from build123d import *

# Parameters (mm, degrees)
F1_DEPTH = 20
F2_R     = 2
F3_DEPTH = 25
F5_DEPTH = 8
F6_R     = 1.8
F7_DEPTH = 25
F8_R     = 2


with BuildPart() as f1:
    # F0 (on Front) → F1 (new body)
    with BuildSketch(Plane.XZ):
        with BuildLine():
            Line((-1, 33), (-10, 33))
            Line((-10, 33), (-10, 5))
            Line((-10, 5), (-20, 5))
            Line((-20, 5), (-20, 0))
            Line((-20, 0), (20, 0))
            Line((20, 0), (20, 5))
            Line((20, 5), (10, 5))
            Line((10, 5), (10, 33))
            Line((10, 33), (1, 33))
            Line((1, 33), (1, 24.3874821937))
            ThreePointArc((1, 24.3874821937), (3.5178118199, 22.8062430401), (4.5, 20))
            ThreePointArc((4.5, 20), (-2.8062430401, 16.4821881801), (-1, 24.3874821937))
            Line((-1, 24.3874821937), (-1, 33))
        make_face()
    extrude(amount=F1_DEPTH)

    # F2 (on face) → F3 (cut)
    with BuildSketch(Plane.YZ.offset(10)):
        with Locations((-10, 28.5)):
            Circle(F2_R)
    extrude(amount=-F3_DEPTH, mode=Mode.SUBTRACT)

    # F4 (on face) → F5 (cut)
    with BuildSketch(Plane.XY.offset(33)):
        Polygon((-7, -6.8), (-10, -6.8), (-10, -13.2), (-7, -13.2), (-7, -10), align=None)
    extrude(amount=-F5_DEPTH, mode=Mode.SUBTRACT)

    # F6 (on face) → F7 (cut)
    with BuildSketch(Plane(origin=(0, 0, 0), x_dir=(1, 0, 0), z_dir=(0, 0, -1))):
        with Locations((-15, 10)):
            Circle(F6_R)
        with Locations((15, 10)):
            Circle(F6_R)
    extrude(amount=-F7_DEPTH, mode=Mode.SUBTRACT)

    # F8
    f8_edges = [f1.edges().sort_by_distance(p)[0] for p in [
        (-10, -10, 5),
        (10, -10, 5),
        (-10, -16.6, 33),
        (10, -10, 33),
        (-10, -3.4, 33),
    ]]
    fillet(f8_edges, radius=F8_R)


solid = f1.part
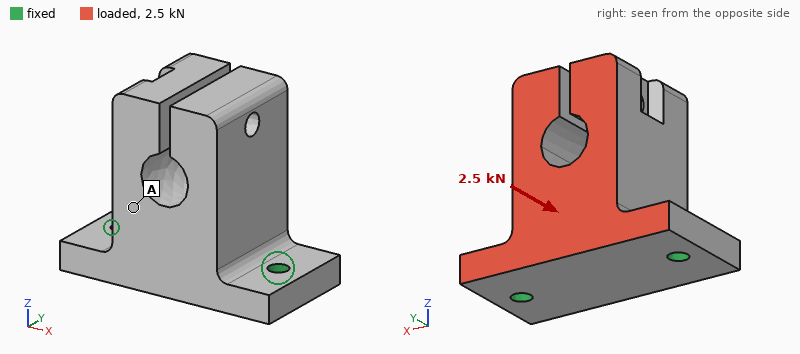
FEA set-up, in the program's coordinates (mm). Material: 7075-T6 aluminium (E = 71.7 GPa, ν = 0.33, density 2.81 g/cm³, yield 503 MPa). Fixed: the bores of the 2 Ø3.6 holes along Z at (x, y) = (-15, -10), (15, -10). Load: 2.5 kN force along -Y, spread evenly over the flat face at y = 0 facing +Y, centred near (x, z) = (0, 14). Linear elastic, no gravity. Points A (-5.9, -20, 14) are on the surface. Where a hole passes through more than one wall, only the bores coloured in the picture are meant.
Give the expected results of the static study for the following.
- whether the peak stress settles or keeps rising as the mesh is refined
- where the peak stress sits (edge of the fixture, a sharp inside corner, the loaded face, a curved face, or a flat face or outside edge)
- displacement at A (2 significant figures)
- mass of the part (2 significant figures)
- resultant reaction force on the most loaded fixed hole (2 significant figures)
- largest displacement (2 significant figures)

keeps rising
edge of the fixture
0.072 mm
37 g
1.3 kN
0.15 mm
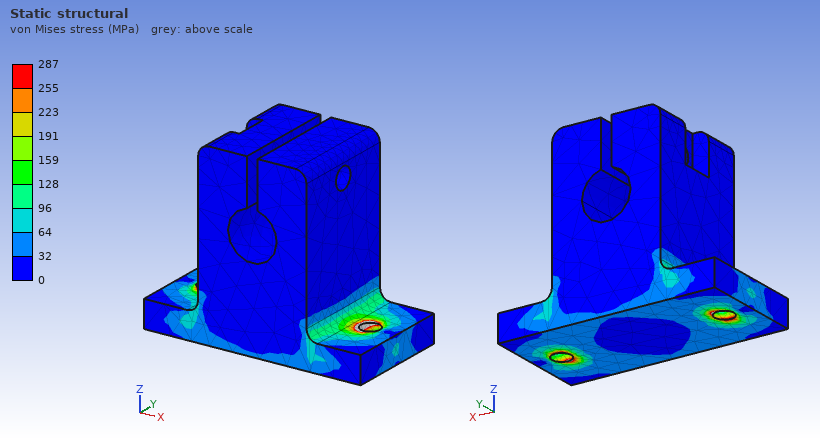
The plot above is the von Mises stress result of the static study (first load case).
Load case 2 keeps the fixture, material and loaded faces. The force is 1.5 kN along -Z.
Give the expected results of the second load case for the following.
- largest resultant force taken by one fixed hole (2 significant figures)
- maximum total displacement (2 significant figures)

800 N
76 µm
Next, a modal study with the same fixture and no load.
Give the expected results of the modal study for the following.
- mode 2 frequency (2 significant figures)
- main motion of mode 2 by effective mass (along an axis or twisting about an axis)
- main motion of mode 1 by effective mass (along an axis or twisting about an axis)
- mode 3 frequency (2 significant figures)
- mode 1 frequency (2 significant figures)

8100 Hz
along X
along Y
10 kHz
4100 Hz
